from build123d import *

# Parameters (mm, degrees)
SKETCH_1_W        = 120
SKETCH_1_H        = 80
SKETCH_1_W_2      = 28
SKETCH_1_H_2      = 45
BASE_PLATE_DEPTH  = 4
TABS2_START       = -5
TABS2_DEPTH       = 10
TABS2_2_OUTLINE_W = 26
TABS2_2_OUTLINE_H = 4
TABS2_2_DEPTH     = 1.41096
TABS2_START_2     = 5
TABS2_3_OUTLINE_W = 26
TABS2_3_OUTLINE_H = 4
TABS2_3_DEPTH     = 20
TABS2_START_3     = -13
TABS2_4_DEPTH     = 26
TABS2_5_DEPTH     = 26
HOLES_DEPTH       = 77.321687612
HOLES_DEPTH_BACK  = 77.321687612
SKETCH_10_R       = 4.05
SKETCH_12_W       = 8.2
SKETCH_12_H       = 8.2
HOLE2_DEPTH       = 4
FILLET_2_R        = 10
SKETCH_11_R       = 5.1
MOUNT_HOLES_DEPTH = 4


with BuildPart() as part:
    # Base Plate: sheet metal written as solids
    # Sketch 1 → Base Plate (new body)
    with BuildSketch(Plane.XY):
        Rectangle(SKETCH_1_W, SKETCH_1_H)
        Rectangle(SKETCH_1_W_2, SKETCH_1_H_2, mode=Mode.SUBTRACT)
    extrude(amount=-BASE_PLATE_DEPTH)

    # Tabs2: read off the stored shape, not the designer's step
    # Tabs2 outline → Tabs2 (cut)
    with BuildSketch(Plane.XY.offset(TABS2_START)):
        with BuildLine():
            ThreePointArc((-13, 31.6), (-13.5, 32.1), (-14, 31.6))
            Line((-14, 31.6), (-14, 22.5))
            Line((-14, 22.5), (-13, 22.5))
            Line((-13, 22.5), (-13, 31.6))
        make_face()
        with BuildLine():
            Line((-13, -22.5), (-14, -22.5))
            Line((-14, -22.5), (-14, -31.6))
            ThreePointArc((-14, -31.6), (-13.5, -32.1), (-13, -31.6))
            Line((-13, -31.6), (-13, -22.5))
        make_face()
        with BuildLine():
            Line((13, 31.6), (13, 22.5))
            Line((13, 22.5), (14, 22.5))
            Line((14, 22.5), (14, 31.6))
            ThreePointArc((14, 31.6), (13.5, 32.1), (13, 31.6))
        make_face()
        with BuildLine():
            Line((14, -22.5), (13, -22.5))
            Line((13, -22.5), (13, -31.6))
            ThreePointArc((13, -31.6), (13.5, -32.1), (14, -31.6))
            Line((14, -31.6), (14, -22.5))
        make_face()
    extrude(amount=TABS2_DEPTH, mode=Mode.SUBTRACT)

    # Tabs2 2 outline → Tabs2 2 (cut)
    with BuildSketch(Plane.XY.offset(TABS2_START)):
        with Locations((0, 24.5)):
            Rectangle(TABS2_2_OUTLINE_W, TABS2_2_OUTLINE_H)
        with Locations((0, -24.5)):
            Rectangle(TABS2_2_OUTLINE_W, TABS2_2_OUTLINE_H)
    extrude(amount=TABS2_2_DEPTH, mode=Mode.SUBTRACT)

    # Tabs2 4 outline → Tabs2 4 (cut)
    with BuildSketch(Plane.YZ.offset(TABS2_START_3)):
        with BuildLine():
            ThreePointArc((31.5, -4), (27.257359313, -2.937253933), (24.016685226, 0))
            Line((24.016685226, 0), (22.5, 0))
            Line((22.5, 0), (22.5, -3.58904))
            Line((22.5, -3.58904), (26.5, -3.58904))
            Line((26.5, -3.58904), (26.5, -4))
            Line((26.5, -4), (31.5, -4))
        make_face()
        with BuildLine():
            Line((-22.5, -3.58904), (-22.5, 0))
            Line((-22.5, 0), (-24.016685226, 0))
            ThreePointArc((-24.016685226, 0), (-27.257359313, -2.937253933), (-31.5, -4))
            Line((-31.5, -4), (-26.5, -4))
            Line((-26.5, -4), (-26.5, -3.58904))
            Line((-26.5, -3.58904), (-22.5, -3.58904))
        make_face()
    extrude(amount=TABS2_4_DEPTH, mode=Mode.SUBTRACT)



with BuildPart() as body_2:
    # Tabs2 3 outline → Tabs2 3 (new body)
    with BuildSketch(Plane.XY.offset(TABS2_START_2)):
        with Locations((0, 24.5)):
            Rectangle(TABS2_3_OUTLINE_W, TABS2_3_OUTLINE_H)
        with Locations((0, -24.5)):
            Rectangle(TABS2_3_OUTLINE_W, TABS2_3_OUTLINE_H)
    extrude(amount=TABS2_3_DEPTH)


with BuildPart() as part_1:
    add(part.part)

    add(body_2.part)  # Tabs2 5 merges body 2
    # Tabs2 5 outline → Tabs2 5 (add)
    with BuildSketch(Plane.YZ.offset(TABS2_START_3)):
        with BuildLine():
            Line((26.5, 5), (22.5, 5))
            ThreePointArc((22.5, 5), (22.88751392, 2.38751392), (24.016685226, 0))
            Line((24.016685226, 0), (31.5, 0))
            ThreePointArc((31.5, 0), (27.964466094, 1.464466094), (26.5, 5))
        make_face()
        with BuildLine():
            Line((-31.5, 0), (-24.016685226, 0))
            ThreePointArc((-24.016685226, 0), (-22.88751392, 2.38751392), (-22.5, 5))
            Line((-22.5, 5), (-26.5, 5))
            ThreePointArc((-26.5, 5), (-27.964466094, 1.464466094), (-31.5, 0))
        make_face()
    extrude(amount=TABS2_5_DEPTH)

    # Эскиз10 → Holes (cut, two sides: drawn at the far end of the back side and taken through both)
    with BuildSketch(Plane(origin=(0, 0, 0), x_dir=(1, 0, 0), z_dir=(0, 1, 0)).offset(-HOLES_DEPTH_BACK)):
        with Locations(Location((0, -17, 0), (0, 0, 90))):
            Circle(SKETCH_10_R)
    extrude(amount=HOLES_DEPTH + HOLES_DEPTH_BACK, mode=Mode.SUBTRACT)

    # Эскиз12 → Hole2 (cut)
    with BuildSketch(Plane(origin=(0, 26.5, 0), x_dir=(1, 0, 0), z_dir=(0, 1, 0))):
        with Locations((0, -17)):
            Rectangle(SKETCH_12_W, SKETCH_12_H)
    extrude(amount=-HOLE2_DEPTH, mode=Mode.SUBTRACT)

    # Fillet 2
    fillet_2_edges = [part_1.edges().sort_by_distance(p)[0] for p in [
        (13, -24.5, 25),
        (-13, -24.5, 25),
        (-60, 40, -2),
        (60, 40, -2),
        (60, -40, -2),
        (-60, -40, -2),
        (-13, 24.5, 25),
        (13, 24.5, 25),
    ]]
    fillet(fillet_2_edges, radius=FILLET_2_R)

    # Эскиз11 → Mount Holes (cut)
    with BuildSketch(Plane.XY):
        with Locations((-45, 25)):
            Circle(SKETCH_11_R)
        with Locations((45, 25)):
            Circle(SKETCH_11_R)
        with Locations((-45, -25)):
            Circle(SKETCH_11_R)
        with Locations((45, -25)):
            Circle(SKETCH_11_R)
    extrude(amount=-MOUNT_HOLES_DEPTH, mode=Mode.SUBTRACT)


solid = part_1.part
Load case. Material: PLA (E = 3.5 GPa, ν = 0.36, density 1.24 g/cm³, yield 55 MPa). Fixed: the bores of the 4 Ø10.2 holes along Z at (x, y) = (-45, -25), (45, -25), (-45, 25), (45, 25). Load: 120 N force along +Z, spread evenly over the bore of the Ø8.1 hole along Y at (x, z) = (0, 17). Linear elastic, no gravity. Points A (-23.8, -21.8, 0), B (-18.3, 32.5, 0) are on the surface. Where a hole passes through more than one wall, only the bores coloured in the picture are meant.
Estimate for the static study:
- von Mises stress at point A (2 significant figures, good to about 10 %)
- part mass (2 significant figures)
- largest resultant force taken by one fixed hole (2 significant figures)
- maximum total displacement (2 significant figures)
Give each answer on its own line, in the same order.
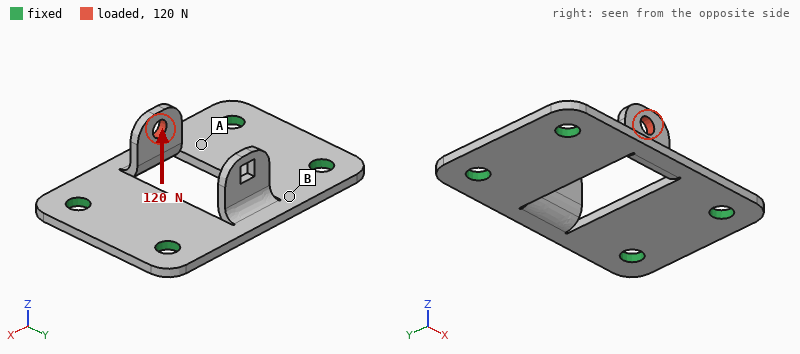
5.6 MPa
44 g
60 N
1.7 mm
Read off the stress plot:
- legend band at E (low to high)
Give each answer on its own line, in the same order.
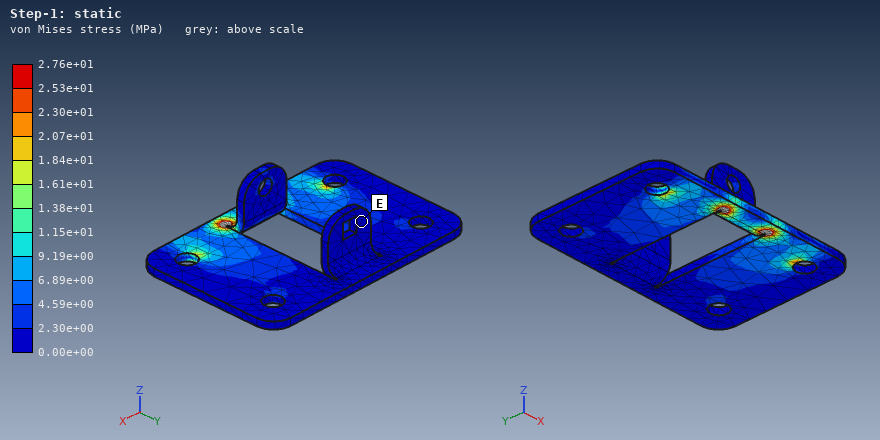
0.00e+00 to 2.30e+00 MPa
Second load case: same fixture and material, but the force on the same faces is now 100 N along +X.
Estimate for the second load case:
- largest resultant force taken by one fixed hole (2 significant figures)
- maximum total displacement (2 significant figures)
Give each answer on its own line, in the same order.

81 N
0.85 mm
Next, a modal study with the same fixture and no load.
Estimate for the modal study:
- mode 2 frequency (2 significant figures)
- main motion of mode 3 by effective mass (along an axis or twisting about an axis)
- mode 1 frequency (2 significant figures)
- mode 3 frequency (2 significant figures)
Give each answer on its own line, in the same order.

710 Hz
along Z
670 Hz
910 Hz
